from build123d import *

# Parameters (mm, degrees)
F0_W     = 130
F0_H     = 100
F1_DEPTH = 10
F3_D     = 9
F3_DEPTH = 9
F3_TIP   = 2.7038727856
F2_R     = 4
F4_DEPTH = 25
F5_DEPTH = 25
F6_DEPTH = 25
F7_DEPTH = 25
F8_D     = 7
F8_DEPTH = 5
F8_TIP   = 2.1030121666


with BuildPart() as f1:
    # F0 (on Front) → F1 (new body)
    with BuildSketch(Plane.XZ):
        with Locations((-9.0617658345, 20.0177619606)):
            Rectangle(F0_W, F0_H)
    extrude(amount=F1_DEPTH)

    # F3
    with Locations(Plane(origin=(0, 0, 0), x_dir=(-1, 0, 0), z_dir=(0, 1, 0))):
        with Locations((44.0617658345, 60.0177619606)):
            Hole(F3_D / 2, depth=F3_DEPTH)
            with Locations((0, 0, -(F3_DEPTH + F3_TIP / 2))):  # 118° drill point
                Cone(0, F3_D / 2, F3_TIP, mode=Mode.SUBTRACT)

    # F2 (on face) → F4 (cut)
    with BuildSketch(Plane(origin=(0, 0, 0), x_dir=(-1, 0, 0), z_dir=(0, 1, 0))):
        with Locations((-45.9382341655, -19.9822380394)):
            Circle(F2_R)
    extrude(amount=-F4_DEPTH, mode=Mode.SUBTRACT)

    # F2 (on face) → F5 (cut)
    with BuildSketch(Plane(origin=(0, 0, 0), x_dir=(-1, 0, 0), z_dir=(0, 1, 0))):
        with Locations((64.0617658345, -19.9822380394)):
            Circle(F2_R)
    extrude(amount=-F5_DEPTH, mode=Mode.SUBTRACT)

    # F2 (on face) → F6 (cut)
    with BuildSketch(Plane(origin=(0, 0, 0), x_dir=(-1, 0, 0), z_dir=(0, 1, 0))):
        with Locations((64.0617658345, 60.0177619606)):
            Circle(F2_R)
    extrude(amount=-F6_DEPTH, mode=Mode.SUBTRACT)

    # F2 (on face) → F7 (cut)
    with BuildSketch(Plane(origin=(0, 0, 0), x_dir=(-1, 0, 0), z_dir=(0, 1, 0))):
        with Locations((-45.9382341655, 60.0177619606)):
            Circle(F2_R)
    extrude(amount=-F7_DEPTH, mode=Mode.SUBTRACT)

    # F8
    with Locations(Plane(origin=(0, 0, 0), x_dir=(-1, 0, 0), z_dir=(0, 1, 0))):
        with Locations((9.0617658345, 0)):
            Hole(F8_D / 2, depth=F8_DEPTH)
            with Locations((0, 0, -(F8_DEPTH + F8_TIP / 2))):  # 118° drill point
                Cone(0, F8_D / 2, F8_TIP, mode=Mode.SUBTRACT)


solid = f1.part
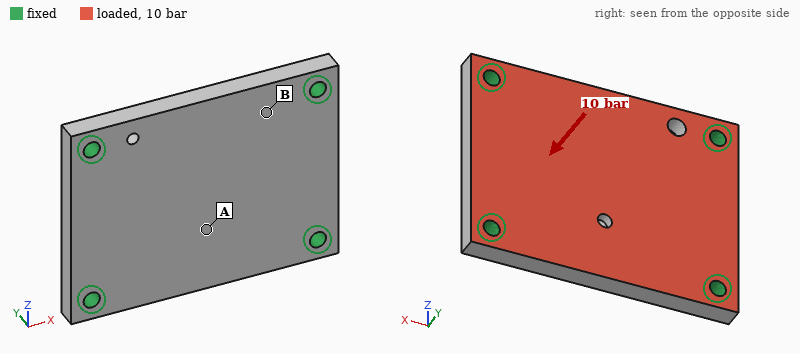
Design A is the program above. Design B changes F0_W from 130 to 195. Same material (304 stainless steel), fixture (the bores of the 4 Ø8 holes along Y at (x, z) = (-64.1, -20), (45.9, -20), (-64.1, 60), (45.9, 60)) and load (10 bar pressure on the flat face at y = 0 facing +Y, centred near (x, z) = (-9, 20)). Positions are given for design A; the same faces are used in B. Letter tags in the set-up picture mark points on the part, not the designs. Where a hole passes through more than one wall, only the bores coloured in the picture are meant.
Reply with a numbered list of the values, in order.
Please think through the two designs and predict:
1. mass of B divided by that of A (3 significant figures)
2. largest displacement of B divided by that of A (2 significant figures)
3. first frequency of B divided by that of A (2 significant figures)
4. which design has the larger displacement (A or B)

1. 1.51
2. 0.88
3. 0.93
4. A
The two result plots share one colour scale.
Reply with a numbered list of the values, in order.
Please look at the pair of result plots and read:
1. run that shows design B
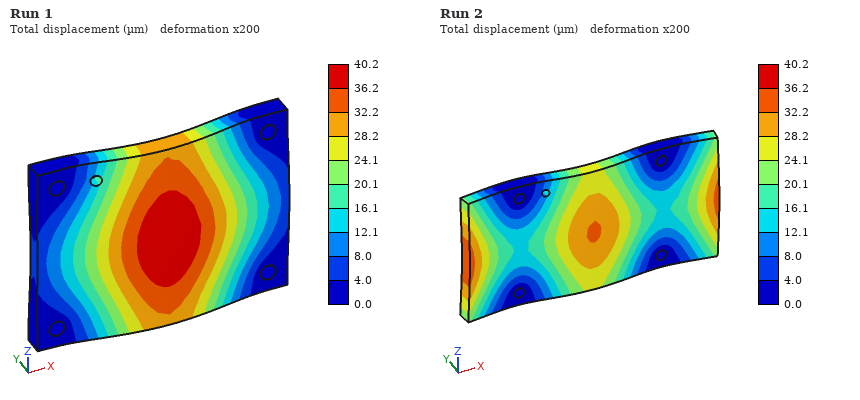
1. Run 2
